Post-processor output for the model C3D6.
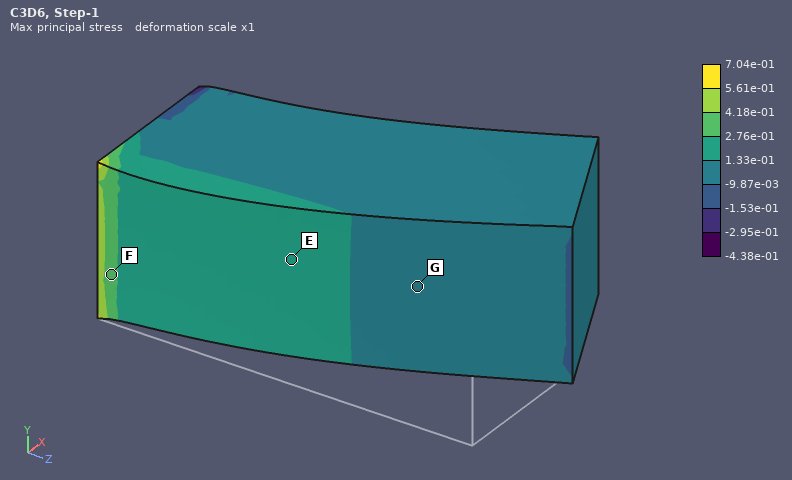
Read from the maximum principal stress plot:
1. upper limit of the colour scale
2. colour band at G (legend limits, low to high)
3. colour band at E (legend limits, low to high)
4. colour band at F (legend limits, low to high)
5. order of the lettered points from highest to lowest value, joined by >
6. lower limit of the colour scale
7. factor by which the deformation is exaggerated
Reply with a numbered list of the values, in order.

1. 7.04e-01
2. -9.87e-03 to 1.33e-01
3. 1.33e-01 to 2.76e-01
4. 2.76e-01 to 4.18e-01
5. F > E > G
6. -4.38e-01
7. 1
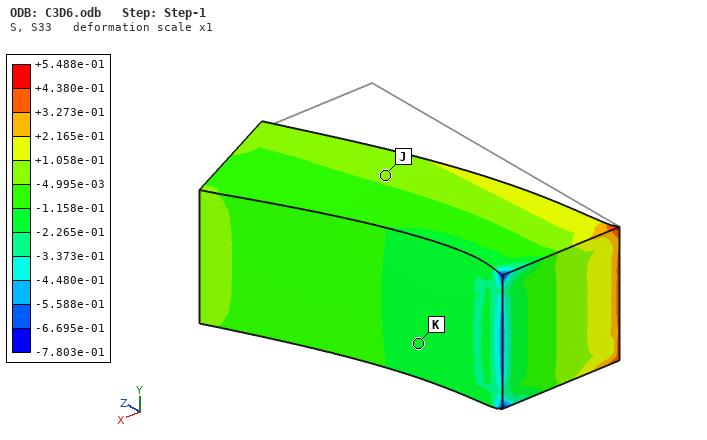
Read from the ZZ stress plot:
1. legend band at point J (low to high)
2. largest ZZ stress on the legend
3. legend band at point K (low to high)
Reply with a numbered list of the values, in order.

1. -4.995e-03 to +1.058e-01
2. +5.488e-01
3. -2.265e-01 to -1.158e-01
